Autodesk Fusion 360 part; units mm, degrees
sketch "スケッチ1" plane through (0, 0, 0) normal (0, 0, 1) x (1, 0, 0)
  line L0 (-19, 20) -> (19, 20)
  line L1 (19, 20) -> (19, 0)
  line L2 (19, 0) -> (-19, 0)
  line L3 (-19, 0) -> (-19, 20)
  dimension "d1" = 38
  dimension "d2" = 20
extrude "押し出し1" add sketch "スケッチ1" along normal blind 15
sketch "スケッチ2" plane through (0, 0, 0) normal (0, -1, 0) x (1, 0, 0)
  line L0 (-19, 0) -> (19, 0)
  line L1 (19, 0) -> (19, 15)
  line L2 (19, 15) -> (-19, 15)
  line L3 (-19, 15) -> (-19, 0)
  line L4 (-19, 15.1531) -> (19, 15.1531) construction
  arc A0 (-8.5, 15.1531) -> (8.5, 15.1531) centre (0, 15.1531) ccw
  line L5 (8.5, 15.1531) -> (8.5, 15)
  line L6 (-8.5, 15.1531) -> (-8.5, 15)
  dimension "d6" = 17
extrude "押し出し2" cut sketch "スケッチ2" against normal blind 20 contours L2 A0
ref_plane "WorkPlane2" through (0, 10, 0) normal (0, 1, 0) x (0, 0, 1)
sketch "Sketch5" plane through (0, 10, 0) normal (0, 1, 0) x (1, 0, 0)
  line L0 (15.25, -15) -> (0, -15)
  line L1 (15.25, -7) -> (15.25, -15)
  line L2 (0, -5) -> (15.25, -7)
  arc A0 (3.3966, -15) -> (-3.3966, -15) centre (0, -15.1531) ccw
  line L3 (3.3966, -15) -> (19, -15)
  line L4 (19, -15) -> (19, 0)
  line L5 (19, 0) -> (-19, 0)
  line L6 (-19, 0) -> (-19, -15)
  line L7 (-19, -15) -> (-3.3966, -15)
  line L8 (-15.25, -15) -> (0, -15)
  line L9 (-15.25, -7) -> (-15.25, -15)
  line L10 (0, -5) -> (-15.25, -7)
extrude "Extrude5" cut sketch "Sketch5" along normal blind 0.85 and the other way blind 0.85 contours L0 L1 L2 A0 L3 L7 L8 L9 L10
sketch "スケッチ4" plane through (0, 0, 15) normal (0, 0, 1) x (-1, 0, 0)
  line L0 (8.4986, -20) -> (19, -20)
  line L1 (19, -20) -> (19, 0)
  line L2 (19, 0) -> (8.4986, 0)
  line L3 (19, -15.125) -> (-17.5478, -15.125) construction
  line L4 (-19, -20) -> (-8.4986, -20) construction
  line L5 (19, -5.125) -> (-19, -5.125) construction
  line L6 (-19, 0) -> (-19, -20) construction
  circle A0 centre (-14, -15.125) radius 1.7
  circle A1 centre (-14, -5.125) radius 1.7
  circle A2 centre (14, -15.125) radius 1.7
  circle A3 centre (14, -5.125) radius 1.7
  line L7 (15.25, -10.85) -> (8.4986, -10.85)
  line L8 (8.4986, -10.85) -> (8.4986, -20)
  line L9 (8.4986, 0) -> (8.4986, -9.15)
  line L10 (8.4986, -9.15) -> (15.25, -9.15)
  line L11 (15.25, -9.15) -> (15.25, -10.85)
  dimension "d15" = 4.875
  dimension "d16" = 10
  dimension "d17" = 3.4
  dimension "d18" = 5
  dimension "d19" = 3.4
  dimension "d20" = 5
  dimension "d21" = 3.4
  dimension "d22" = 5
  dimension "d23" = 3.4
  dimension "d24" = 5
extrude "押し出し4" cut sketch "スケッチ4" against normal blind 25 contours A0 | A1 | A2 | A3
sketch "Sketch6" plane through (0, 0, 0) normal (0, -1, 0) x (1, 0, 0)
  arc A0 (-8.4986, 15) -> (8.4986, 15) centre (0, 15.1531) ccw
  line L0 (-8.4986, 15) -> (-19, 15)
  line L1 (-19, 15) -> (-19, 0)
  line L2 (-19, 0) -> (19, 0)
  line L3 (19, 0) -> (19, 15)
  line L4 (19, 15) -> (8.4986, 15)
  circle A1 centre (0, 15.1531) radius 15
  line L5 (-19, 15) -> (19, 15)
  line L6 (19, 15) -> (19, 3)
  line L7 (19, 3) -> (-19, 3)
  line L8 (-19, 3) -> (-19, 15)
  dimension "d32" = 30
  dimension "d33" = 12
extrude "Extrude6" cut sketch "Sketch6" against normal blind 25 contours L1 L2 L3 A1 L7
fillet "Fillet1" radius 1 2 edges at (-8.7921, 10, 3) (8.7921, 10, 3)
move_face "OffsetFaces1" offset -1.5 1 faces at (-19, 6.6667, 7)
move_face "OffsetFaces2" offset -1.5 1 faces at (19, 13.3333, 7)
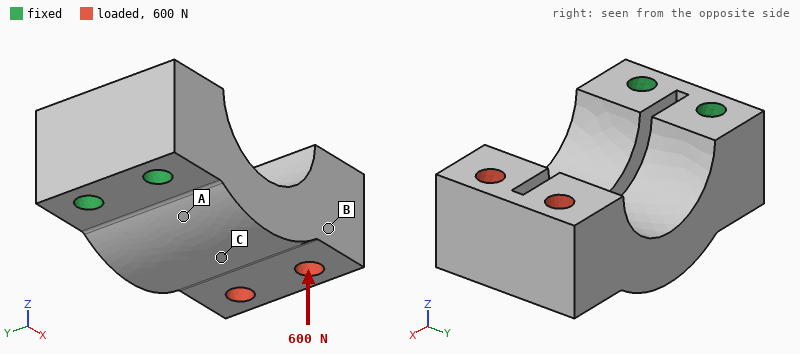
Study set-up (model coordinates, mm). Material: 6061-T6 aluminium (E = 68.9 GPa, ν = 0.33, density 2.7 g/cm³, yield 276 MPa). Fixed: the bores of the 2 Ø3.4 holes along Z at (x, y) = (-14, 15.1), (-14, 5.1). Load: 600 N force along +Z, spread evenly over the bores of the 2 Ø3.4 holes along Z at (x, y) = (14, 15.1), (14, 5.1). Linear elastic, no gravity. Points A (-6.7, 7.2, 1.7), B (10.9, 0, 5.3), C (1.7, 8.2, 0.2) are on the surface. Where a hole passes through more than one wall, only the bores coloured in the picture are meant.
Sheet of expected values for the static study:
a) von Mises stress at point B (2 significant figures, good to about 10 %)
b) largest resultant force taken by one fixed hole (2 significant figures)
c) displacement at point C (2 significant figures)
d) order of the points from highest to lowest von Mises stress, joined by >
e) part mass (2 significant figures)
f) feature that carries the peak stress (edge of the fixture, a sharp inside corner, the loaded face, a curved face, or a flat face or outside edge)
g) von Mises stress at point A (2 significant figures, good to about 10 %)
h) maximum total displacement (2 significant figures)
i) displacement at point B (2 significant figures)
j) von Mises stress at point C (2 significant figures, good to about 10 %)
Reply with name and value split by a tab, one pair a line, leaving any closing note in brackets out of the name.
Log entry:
von Mises stress at point B	15 MPa
largest resultant force taken by one fixed hole	340 N
displacement at point C	0.040 mm
order of the points from highest to lowest von Mises stress, joined by >	A > C > B
part mass	17 g
feature that carries the peak stress	a curved face
von Mises stress at point A	65 MPa
maximum total displacement	0.14 mm
displacement at point B	0.083 mm
von Mises stress at point C	44 MPa
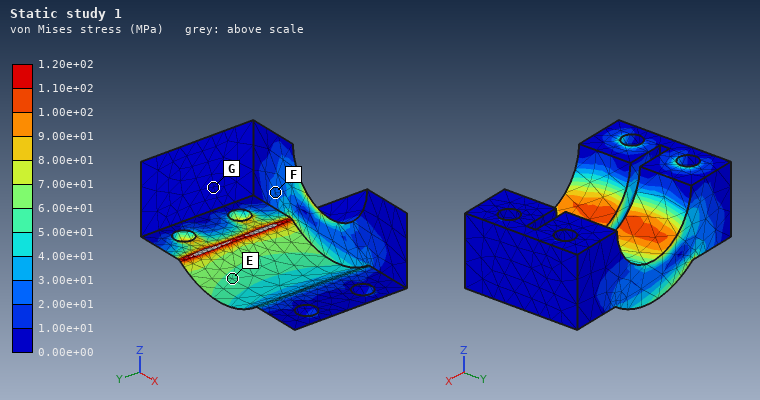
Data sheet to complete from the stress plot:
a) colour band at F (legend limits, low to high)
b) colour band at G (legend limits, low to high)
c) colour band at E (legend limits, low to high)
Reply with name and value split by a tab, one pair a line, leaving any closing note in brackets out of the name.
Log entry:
colour band at F	2.00e+01 to 3.00e+01 MPa
colour band at G	0.00e+00 to 1.00e+01 MPa
colour band at E	5.00e+01 to 6.00e+01 MPa
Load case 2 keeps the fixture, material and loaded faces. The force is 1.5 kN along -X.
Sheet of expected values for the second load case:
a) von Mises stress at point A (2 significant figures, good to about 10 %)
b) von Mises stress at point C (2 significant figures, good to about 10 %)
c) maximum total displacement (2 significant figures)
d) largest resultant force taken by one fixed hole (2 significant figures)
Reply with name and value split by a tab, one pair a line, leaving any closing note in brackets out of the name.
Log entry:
von Mises stress at point A	29 MPa
von Mises stress at point C	36 MPa
maximum total displacement	90 µm
largest resultant force taken by one fixed hole	760 N
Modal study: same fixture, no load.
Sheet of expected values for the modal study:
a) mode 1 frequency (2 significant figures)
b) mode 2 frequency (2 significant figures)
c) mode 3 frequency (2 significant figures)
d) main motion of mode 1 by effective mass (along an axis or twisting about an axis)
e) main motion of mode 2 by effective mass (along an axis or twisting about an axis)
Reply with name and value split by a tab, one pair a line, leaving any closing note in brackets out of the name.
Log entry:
mode 1 frequency	5000 Hz
mode 2 frequency	8000 Hz
mode 3 frequency	15 kHz
main motion of mode 1 by effective mass	along Z
main motion of mode 2 by effective mass	along Y
